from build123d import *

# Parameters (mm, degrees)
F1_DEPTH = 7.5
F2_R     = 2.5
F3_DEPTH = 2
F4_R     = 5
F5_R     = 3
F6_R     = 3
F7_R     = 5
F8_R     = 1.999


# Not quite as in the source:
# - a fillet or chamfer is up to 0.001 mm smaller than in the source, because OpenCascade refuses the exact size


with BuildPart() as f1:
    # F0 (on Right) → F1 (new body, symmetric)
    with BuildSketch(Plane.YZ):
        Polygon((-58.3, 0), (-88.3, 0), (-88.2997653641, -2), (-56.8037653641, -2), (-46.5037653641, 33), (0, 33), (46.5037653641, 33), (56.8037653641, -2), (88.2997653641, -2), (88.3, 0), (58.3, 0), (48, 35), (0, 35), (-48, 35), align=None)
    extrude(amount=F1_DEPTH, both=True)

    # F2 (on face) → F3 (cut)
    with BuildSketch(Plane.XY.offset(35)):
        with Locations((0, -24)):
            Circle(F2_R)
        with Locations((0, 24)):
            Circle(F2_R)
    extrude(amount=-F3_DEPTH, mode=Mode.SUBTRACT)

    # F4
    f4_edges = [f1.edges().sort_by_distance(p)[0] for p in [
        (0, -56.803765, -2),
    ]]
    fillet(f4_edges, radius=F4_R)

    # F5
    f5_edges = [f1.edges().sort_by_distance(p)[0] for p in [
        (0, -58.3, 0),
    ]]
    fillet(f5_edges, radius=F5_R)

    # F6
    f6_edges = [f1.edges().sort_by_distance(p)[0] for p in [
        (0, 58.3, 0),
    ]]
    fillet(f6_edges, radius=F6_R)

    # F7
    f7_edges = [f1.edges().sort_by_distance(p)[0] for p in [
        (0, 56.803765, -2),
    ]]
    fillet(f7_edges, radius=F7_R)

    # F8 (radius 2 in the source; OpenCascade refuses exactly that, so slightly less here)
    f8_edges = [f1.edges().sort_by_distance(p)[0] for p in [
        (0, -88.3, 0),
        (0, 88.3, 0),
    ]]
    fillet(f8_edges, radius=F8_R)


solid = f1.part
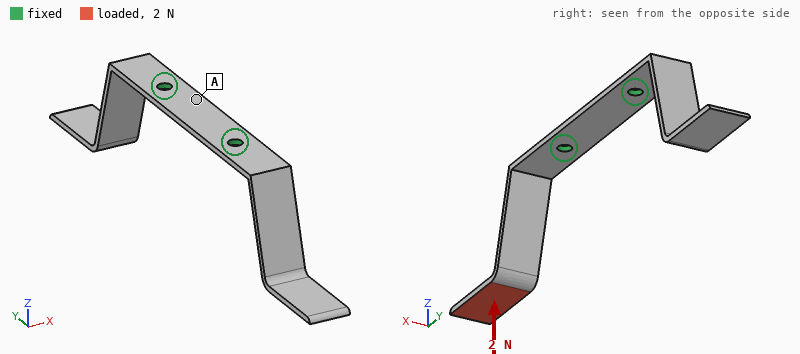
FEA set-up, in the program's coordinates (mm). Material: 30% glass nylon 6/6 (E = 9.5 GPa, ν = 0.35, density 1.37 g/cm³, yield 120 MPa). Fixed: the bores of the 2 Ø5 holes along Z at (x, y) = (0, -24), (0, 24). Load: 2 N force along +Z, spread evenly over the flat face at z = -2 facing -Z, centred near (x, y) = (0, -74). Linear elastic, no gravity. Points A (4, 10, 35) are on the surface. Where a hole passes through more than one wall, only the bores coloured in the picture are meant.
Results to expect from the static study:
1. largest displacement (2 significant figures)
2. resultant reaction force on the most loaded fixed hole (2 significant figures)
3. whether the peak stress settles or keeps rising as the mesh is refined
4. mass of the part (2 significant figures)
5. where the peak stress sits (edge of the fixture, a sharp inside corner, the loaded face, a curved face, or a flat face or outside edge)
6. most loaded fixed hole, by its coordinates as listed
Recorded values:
1.8 mm
2.0 N
keeps rising
9.2 g
edge of the fixture
(0, -24)
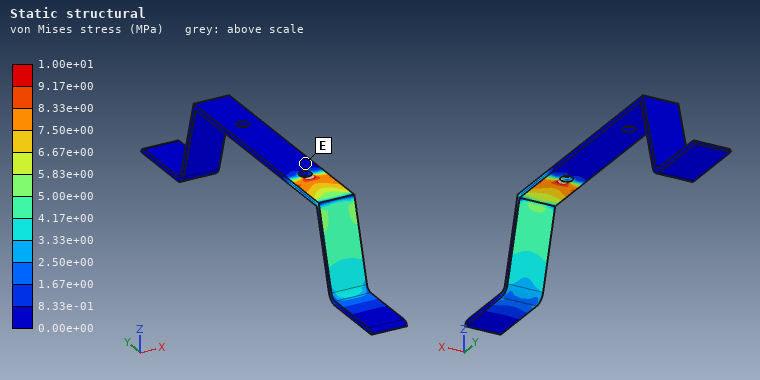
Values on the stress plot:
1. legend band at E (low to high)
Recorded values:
0.00e+00 to 8.33e-01 MPa
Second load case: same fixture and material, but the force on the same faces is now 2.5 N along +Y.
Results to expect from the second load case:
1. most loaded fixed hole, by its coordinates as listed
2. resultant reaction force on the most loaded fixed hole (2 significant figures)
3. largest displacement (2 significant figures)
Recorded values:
(0, -24)
2.4 N
2.0 mm
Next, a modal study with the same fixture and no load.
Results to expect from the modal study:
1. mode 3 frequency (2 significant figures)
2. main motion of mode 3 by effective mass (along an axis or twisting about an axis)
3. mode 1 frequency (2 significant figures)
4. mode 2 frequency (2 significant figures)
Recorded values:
270 Hz
along X
140 Hz
140 Hz
